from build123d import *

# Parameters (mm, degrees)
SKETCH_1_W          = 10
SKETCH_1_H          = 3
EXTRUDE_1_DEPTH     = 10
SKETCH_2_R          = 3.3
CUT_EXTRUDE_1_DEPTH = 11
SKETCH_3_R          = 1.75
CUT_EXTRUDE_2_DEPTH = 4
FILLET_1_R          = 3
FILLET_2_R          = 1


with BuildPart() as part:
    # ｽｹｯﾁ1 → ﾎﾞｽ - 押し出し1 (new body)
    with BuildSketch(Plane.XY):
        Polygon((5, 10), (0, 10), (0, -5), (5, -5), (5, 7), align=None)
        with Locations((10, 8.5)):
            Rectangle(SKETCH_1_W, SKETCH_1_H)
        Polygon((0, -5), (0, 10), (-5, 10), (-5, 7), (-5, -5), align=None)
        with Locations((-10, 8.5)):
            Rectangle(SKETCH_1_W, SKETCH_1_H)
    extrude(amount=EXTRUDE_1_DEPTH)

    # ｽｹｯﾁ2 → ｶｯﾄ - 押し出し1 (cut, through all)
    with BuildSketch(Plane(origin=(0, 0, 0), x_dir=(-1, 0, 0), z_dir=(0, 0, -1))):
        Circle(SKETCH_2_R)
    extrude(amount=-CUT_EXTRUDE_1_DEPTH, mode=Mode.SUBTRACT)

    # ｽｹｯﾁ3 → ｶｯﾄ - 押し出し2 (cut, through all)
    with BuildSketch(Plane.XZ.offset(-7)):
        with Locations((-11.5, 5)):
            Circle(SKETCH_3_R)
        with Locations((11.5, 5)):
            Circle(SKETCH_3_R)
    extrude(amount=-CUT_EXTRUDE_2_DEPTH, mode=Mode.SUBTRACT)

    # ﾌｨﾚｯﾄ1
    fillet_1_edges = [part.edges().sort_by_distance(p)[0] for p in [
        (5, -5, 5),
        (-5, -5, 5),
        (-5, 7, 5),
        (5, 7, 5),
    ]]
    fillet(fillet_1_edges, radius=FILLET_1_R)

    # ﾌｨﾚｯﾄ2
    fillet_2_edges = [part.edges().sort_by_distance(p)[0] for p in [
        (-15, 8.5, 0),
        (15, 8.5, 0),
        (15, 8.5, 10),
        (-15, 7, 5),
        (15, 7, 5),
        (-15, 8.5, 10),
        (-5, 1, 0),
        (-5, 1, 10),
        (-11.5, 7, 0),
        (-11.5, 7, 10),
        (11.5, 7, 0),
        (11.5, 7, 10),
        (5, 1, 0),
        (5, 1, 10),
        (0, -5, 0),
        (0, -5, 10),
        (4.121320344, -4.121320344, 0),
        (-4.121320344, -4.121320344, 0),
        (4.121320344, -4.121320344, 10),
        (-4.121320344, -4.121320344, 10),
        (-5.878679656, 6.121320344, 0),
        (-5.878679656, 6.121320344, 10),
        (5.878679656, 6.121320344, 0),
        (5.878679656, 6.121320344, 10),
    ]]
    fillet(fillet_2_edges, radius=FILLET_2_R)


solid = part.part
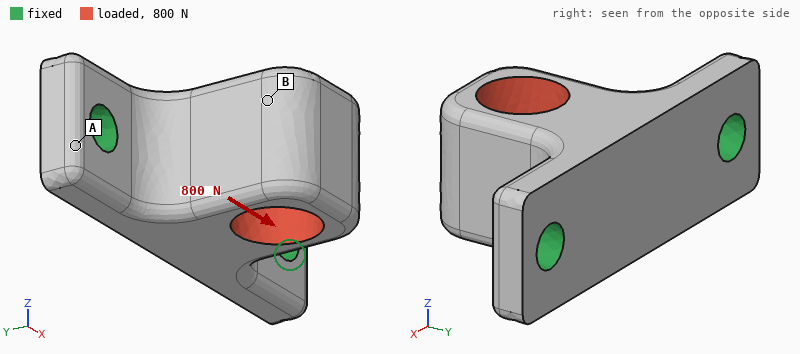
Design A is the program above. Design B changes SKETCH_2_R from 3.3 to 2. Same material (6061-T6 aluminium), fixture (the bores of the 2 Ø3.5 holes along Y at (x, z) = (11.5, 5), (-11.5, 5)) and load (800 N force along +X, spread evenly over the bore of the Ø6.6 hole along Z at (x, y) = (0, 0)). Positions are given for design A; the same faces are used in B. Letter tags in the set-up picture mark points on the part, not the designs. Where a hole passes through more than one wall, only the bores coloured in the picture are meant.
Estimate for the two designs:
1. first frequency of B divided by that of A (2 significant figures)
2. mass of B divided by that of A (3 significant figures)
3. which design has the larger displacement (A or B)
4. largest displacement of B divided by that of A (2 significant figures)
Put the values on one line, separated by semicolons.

0.88; 1.13; A; 0.66
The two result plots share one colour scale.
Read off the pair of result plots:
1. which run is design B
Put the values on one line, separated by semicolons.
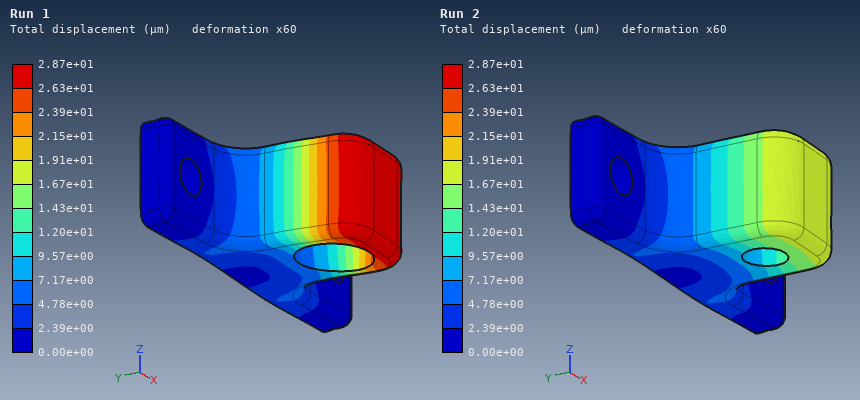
Run 2
